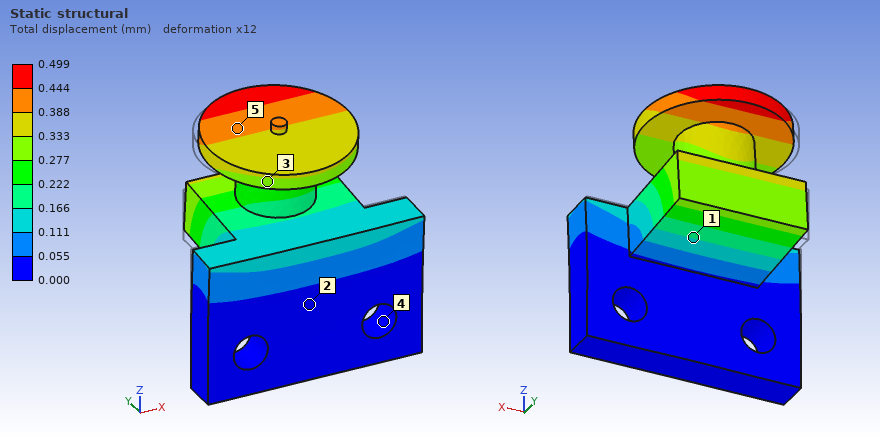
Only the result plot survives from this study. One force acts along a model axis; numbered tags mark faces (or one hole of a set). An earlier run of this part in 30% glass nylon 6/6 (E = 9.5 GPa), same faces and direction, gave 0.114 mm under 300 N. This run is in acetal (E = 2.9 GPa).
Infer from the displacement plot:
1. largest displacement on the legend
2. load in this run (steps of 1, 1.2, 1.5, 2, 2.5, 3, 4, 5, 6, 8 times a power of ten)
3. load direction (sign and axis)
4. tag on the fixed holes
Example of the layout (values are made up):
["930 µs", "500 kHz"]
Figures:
["0.499 mm", "400 N", "+Z", "4"]
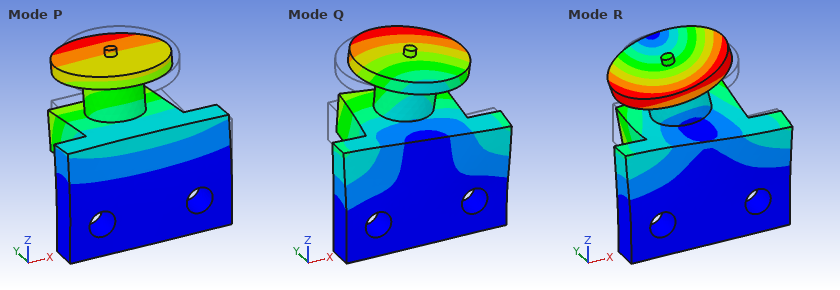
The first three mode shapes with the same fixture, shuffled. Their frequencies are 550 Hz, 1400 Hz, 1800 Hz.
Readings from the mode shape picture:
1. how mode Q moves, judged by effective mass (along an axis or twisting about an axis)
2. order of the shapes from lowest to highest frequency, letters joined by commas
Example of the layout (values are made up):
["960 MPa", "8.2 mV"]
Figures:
["along X", "P, Q, R"]
